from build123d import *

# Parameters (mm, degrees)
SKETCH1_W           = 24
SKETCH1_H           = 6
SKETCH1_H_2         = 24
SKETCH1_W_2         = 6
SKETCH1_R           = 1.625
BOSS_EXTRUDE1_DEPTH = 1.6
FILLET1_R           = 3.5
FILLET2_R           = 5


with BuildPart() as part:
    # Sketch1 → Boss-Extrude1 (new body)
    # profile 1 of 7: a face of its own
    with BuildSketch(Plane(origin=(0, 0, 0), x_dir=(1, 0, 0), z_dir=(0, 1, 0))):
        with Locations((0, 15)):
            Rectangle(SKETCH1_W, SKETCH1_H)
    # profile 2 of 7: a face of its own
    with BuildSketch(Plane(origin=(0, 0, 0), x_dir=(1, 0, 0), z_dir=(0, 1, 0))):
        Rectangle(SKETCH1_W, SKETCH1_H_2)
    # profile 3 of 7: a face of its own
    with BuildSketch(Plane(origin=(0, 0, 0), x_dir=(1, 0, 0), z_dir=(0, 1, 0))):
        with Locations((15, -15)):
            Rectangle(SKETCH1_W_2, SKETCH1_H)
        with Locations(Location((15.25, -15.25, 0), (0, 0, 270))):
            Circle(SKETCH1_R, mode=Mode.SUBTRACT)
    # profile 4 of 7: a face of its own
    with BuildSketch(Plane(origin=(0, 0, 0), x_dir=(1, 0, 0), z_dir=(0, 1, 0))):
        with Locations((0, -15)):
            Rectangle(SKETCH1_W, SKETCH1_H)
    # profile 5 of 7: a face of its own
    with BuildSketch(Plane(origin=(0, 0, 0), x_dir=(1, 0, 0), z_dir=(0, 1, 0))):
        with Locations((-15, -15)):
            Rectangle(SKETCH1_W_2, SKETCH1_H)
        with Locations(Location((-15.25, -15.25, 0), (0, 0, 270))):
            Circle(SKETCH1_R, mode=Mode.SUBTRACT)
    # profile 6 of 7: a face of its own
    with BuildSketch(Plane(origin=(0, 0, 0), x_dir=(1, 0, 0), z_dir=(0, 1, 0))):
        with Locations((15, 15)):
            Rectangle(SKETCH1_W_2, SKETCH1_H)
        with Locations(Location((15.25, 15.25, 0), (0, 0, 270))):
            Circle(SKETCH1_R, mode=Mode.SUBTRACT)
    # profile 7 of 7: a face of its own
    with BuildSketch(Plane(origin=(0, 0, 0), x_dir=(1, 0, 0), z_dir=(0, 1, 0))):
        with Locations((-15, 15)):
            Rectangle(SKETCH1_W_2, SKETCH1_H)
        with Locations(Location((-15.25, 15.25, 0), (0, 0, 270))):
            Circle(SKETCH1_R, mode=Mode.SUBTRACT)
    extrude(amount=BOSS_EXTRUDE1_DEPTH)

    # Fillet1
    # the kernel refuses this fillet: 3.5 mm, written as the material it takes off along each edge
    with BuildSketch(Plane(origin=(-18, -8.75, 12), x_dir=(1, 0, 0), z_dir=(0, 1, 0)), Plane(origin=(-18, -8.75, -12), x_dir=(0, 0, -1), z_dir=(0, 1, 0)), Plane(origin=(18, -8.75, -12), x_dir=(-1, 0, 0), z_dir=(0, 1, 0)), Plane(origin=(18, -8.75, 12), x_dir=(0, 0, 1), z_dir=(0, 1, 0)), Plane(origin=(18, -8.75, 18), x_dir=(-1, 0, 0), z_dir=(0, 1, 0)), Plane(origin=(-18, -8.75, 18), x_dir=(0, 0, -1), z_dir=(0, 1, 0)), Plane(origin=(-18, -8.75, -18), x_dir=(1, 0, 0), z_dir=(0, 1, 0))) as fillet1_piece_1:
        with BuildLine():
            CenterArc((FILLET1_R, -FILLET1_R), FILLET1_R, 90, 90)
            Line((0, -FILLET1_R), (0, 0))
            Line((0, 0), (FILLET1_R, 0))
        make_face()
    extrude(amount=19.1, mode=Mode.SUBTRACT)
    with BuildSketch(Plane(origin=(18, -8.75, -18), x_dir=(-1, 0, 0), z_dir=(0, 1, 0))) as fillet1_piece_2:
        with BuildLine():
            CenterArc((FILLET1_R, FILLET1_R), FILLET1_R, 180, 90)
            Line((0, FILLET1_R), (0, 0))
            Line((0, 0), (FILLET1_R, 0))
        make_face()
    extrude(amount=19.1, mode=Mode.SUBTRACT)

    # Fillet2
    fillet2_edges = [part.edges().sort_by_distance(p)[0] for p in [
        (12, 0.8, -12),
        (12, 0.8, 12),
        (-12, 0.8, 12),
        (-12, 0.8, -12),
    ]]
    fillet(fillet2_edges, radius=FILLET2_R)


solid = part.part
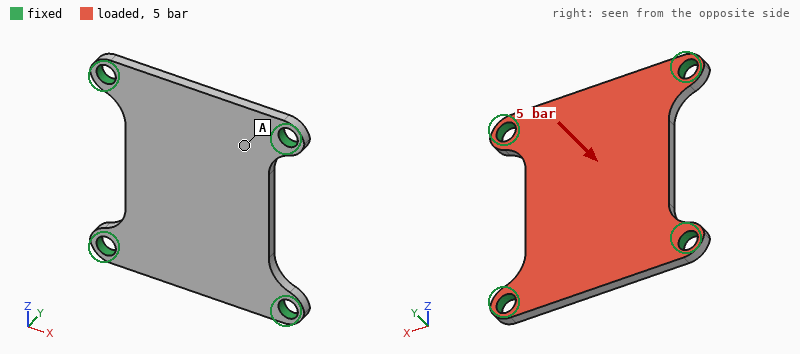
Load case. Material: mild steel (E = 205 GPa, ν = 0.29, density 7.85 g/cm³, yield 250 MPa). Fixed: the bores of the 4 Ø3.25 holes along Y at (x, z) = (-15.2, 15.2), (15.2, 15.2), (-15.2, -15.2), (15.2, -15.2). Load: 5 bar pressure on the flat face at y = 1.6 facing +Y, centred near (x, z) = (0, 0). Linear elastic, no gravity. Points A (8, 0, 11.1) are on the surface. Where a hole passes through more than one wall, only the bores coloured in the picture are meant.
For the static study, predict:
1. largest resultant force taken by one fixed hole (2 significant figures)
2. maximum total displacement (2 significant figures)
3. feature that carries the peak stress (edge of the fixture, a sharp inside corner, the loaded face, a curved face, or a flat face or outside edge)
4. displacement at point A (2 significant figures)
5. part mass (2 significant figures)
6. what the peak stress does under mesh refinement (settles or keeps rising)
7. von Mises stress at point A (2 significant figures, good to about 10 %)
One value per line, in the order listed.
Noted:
120 N
39 µm
edge of the fixture
17 µm
12 g
keeps rising
28 MPa
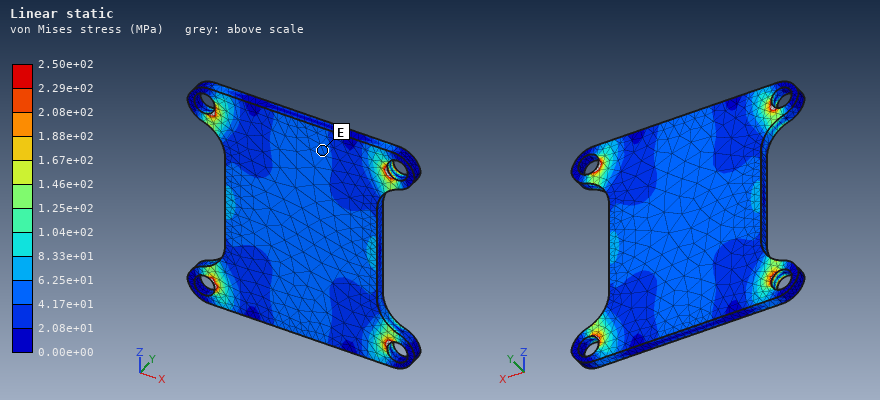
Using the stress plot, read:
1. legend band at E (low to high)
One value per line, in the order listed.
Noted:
4.17e+01 to 6.25e+01 MPa
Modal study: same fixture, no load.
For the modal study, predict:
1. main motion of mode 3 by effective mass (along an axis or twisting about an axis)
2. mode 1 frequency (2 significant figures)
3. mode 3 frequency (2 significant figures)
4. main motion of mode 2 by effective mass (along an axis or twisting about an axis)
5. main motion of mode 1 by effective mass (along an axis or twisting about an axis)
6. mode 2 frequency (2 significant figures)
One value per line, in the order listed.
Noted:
twisting about Z
6100 Hz
12 kHz
twisting about X
along Y
11 kHz
